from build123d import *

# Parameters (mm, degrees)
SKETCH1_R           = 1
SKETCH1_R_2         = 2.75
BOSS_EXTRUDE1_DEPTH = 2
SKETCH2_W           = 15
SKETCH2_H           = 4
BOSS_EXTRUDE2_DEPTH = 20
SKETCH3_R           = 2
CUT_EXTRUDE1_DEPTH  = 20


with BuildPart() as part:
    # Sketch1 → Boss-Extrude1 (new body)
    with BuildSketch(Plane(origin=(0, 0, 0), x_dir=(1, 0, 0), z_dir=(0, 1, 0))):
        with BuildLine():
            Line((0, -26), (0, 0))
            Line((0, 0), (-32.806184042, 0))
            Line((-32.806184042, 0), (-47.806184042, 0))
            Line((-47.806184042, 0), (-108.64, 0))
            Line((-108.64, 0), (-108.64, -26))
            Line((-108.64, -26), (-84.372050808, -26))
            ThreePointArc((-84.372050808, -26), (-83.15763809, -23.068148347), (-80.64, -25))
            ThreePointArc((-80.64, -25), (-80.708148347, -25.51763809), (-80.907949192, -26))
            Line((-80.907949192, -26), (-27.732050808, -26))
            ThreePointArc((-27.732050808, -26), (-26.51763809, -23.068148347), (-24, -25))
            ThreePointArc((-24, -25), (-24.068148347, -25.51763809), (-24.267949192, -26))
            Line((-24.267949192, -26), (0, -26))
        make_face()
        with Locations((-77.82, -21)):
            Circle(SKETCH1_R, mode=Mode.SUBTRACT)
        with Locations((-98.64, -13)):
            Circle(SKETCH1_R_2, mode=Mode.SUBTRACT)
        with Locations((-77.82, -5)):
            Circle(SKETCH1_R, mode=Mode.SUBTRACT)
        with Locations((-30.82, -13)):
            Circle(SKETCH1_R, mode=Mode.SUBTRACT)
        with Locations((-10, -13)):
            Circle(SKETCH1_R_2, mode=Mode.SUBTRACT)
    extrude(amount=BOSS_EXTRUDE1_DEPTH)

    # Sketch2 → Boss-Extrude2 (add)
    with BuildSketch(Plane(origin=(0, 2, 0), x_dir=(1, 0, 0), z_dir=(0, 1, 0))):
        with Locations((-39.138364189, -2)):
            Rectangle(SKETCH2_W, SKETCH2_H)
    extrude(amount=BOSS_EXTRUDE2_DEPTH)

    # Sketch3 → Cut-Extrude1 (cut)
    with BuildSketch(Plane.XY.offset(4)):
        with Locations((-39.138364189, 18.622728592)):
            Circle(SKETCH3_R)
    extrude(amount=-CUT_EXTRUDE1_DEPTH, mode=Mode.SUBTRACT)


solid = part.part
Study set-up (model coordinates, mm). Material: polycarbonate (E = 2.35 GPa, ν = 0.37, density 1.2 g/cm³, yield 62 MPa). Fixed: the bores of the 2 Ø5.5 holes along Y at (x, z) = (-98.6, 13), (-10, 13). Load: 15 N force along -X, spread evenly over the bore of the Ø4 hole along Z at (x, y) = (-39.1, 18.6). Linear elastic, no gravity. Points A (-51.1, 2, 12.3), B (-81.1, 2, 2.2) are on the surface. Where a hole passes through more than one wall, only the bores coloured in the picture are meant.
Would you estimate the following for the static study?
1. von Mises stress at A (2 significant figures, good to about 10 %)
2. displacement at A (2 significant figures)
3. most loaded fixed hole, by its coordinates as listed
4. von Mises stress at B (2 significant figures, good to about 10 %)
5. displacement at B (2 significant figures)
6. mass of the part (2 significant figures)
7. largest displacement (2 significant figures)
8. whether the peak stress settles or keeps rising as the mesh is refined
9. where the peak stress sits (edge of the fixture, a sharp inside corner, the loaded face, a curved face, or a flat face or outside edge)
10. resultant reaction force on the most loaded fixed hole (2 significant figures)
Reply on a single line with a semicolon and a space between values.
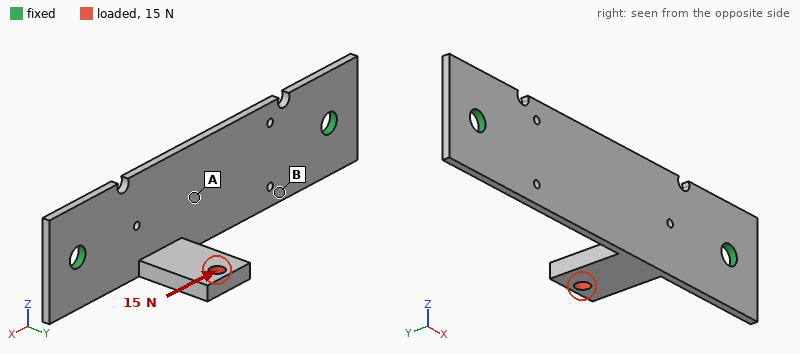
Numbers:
5.3 MPa; 0.60 mm; (-10, 13); 2.1 MPa; 0.29 mm; 8.0 g; 1.1 mm; keeps rising; a sharp inside corner; 11 N
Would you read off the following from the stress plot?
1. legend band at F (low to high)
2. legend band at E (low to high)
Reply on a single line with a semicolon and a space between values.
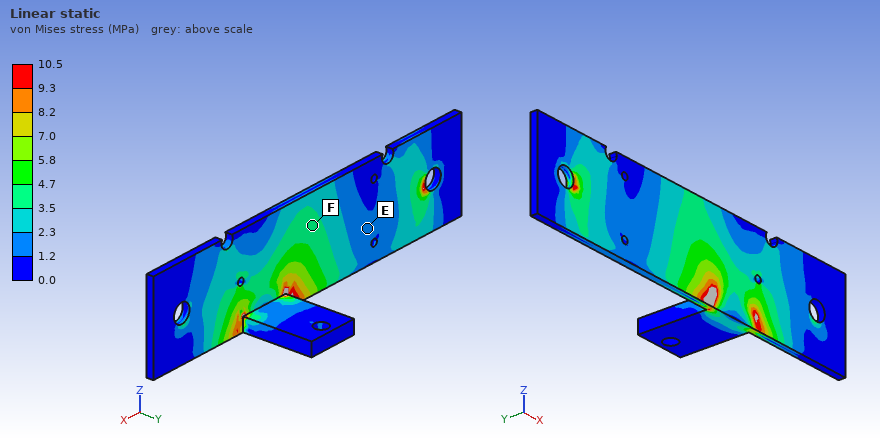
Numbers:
3.5 to 4.7 MPa; 1.2 to 2.3 MPa
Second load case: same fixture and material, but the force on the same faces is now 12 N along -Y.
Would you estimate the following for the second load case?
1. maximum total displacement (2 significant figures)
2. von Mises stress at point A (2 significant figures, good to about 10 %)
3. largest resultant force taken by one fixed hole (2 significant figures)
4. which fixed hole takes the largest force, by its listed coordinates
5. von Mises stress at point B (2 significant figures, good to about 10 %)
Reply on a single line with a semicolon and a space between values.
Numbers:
1.3 mm; 4.0 MPa; 9.0 N; (-10, 13); 2.8 MPa
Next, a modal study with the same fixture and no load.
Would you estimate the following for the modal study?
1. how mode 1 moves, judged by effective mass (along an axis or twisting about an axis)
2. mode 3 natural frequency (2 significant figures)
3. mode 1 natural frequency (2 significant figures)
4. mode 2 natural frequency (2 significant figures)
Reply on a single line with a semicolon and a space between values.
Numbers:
along Y; 910 Hz; 320 Hz; 460 Hz
